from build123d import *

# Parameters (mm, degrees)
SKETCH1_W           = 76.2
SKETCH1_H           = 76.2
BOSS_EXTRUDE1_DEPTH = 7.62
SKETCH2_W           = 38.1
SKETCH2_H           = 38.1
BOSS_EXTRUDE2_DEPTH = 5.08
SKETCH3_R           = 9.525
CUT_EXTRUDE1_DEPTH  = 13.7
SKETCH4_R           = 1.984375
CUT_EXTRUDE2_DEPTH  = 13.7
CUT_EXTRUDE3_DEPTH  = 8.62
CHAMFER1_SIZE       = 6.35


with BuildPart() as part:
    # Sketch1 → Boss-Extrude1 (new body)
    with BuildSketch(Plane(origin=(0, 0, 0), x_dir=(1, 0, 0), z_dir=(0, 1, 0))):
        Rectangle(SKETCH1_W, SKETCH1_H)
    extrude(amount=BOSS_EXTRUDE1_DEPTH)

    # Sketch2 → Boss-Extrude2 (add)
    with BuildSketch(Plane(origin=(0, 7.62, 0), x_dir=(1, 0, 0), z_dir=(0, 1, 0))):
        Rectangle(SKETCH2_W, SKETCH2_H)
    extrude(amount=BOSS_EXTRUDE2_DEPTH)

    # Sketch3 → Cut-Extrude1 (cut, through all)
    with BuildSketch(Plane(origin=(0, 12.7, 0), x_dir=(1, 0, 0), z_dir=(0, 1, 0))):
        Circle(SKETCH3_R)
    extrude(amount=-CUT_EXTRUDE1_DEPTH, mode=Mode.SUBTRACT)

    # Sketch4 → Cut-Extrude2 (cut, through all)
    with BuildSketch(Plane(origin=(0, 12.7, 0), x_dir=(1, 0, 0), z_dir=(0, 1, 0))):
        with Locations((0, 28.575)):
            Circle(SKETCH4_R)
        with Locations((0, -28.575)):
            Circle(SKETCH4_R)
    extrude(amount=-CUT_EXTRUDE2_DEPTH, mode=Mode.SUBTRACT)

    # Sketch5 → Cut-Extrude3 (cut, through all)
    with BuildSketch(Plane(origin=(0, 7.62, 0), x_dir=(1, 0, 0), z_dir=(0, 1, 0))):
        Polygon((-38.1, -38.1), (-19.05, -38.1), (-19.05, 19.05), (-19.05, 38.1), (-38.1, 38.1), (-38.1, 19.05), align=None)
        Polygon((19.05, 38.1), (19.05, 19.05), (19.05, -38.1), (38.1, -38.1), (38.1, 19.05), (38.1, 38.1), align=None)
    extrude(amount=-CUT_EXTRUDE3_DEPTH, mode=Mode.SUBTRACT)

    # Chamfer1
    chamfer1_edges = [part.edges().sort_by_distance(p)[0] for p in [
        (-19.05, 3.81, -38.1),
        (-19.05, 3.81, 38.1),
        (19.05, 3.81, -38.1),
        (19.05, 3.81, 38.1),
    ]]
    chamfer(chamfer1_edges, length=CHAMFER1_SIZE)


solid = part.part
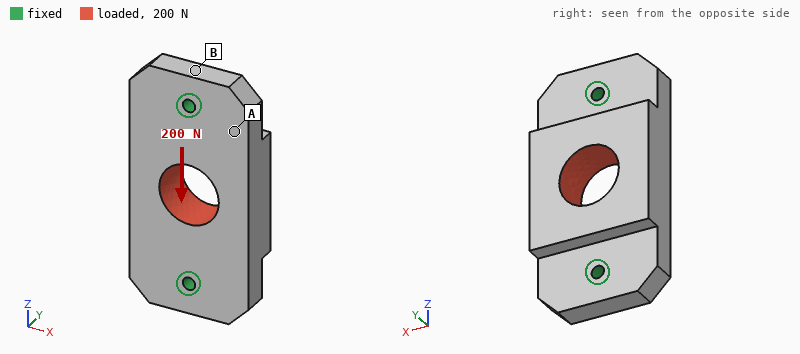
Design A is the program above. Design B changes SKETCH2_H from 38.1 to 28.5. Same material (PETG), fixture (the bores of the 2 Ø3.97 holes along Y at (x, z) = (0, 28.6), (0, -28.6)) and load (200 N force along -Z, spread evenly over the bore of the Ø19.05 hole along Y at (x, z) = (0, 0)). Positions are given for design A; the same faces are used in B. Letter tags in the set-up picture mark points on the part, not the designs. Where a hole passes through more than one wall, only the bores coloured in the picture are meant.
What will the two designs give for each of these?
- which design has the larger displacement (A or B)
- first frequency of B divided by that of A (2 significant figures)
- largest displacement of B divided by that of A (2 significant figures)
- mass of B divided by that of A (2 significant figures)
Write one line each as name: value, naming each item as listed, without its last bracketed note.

which design has the larger displacement: B
first frequency of B divided by that of A: 1.0
largest displacement of B divided by that of A: 1.3
mass of B divided by that of A: 0.93
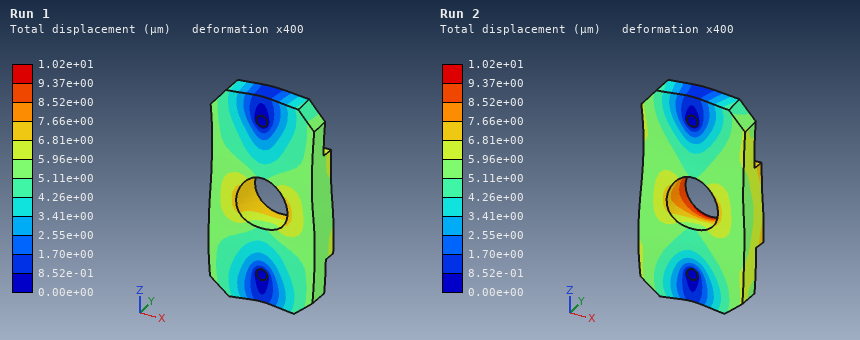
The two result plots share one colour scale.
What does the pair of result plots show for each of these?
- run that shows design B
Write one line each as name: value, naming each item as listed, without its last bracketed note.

run that shows design B: Run 2
